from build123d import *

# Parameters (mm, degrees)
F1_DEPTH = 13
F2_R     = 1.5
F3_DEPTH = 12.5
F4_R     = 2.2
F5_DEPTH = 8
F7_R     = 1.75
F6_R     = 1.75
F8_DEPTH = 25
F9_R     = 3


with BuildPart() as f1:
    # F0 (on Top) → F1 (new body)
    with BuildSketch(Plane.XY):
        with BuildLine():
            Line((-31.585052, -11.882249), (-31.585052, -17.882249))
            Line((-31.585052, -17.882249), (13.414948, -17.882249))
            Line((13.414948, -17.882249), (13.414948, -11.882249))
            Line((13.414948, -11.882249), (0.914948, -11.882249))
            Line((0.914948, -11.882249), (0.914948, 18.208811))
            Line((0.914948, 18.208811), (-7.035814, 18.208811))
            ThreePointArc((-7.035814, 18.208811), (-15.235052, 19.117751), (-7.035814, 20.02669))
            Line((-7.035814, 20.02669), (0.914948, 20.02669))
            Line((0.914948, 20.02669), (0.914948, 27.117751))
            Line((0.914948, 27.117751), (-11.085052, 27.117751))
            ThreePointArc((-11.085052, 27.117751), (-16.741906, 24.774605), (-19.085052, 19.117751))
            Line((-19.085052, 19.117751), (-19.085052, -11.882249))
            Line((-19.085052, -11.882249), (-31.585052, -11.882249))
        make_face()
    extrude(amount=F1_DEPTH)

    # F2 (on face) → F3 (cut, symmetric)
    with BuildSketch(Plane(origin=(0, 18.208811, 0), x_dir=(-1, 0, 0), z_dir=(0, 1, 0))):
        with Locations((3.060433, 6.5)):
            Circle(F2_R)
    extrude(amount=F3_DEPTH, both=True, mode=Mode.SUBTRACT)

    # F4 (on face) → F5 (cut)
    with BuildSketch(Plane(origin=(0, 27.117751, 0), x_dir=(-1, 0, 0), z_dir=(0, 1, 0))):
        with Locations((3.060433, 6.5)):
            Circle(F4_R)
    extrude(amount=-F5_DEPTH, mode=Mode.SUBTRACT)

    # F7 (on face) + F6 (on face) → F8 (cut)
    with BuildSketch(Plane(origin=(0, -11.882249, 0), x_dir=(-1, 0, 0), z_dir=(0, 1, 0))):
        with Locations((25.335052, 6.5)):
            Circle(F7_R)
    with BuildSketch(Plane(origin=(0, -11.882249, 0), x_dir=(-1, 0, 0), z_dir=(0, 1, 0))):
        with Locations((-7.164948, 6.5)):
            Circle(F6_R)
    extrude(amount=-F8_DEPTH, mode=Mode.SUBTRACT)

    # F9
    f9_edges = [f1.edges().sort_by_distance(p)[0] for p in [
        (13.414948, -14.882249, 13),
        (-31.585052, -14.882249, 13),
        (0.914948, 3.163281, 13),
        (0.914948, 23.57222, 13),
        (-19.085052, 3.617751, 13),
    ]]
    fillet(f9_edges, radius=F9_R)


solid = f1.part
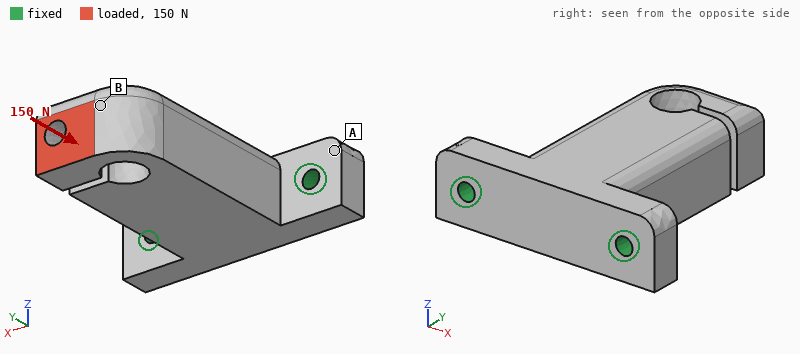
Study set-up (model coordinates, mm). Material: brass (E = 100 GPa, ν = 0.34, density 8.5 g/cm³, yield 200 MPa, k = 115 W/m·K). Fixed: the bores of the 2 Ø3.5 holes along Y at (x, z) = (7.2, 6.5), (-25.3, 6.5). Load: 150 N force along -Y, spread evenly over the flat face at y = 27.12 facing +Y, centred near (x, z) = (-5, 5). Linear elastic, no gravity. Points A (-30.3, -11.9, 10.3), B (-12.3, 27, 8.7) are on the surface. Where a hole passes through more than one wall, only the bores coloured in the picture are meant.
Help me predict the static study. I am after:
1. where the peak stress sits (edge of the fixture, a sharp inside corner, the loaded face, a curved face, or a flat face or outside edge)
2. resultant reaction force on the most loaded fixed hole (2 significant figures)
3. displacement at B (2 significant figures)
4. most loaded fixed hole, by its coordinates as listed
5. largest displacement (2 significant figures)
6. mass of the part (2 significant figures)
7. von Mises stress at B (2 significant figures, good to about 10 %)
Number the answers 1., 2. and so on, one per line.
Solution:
1. a curved face
2. 100 N
3. 26 µm
4. (7.2, 6.5)
5. 69 µm
6. 100 g
7. 27 MPa
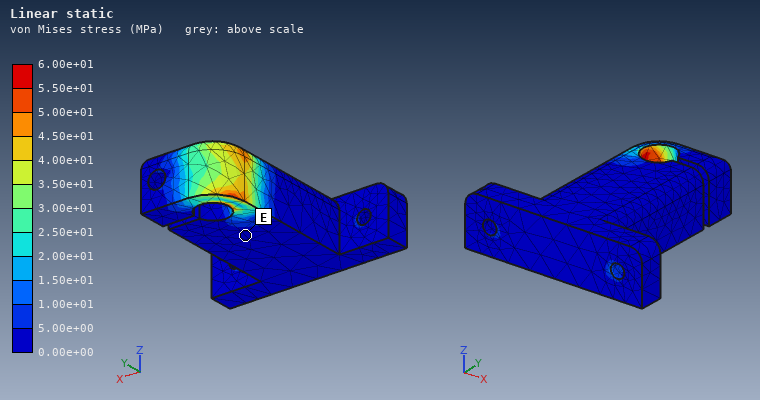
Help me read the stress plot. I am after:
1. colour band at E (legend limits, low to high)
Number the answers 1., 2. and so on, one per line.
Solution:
1. 0.00e+00 to 5.00e+00 MPa
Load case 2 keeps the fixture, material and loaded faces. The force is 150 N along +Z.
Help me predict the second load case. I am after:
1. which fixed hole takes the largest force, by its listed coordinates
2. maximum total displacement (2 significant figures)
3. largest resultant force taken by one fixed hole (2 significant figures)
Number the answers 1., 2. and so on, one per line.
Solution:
1. (7.2, 6.5)
2. 79 µm
3. 93 N
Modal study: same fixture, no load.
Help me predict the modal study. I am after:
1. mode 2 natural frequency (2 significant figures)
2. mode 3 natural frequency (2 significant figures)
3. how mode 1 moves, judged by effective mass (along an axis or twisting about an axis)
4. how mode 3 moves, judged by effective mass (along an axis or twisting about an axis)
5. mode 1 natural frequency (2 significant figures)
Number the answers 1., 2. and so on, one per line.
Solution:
1. 3000 Hz
2. 4600 Hz
3. along Z
4. along X
5. 1800 Hz
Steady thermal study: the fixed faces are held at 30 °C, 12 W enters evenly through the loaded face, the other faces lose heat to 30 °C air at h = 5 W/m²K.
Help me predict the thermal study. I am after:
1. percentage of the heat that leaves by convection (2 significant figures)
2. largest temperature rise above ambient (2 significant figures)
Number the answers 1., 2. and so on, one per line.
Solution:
1. 3.1 %
2. 62 K
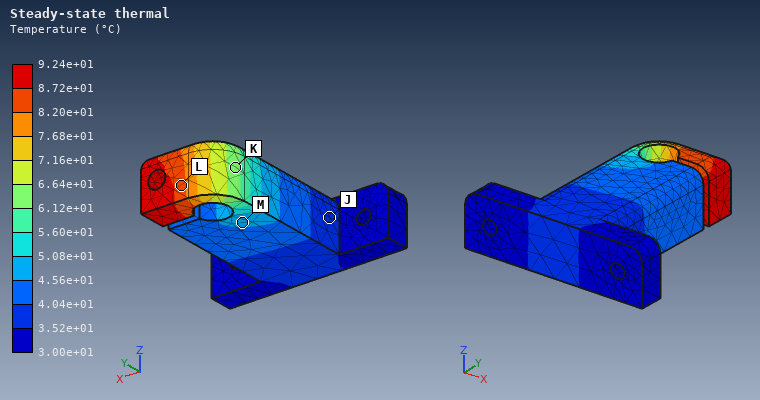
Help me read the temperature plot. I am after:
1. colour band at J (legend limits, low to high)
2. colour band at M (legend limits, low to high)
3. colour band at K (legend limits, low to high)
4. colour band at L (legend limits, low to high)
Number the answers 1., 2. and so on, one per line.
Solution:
1. 3.52e+01 to 4.04e+01 °C
2. 4.56e+01 to 5.08e+01 °C
3. 6.12e+01 to 6.64e+01 °C
4. 8.20e+01 to 8.72e+01 °C
